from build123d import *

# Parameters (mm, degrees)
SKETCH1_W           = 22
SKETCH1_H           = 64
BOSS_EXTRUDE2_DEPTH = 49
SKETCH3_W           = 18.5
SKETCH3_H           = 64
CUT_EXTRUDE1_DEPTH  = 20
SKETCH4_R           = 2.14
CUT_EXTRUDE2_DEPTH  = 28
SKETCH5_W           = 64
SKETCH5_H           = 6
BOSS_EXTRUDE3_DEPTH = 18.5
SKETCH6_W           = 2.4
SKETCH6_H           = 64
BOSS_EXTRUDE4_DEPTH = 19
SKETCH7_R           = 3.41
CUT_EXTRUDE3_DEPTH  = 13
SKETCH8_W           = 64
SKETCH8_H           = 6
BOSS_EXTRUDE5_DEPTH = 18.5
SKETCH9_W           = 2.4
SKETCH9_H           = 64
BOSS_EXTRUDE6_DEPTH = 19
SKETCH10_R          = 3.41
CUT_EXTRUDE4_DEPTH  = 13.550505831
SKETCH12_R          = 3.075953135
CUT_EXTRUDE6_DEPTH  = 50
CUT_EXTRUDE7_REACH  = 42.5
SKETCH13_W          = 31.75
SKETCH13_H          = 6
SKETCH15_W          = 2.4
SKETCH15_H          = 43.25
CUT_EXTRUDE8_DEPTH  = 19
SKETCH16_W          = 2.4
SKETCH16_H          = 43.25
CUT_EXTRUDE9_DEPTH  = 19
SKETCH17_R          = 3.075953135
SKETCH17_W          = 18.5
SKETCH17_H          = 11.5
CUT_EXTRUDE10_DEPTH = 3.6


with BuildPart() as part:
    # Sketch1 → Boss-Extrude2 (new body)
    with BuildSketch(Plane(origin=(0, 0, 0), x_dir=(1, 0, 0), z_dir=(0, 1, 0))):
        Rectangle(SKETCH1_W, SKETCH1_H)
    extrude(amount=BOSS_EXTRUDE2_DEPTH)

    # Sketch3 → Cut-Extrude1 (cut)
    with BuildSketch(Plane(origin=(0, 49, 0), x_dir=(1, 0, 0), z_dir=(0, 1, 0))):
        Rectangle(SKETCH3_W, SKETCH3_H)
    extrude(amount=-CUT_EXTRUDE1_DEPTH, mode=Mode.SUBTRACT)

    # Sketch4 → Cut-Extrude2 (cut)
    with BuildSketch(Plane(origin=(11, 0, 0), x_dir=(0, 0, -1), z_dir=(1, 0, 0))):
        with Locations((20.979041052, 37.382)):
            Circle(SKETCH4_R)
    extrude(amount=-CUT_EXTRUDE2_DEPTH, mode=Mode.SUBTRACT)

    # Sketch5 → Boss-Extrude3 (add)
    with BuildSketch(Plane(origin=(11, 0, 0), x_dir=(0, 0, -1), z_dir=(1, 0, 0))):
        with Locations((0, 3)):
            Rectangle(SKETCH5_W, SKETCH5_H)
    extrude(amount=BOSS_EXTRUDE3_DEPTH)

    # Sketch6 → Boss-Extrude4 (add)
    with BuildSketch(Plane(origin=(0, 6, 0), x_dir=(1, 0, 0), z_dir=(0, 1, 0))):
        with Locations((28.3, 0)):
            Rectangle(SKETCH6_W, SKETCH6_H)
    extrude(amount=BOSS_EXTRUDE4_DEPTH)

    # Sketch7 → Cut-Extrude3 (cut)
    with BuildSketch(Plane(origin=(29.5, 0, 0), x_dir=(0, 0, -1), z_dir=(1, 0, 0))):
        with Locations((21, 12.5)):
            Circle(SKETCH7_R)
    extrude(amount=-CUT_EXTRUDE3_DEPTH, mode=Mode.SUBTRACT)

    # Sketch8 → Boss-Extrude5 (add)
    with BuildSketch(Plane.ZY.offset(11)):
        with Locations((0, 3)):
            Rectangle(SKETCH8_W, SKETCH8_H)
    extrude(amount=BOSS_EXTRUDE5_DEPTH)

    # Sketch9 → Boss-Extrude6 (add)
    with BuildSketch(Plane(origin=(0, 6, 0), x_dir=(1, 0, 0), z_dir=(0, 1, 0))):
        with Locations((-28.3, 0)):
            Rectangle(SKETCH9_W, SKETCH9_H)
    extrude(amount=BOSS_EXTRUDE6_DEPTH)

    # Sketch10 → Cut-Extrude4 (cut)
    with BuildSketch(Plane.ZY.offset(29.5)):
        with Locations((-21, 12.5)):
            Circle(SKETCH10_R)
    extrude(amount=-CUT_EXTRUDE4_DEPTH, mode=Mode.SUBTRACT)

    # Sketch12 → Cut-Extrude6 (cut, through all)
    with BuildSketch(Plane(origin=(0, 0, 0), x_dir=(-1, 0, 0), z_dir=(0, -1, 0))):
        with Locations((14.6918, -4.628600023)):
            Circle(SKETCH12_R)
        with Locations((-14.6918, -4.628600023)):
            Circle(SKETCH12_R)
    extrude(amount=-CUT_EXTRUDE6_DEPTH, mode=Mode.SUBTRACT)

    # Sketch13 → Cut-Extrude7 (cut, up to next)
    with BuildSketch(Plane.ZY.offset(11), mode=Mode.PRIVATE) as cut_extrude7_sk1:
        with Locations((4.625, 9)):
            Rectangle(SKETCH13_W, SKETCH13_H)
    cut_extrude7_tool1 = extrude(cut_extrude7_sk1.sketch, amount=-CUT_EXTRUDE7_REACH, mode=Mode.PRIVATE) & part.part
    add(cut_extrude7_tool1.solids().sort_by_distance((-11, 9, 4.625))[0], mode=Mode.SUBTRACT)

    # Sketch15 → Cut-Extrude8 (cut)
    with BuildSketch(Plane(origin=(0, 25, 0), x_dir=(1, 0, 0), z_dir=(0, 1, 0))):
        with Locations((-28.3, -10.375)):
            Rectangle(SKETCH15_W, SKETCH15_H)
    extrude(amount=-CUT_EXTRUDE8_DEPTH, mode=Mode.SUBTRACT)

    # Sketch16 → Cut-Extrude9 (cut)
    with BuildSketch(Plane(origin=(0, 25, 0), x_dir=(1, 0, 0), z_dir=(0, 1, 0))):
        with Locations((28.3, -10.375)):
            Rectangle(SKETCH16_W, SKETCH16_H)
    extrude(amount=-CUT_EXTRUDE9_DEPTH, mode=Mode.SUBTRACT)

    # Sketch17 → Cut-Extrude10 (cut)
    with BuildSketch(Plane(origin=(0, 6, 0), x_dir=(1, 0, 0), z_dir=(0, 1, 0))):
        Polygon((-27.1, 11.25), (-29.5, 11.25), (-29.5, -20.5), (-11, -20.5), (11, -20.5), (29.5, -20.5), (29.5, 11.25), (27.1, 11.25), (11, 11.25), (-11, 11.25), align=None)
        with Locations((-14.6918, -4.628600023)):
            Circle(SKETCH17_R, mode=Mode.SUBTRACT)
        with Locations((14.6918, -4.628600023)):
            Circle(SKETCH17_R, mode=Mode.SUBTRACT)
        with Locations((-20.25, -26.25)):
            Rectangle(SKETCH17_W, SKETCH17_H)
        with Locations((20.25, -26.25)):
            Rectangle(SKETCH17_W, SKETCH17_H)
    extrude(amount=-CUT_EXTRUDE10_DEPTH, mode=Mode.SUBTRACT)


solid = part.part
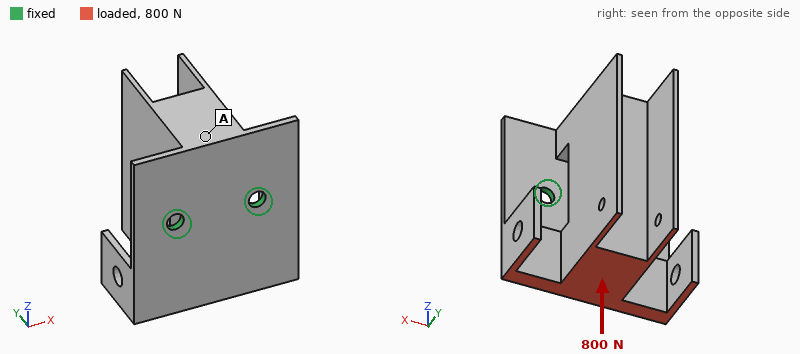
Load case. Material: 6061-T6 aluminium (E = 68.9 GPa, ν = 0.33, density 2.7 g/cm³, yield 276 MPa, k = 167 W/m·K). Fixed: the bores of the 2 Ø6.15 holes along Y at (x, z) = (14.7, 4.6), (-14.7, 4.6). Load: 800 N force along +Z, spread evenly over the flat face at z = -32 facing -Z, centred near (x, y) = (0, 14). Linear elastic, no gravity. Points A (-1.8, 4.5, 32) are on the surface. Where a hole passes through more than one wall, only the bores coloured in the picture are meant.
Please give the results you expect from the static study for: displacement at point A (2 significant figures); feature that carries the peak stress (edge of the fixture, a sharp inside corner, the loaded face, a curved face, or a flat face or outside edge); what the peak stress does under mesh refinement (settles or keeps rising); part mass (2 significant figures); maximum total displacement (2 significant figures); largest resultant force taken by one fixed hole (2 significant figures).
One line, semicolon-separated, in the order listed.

0.15 mm; edge of the fixture; keeps rising; 130 g; 0.32 mm; 400 N
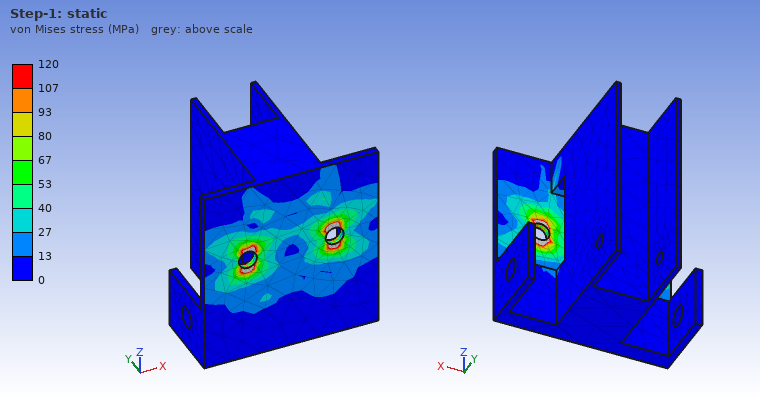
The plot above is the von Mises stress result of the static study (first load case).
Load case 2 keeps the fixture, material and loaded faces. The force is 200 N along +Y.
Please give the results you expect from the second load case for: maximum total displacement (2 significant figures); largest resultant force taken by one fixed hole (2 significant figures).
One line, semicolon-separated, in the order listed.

0.23 mm; 100 N
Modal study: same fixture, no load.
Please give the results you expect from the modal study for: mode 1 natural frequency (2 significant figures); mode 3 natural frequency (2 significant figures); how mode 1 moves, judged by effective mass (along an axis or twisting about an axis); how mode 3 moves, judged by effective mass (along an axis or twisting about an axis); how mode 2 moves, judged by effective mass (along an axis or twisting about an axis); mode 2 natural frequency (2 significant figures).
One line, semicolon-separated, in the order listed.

690 Hz; 2100 Hz; along Z; along Y; along X; 1300 Hz
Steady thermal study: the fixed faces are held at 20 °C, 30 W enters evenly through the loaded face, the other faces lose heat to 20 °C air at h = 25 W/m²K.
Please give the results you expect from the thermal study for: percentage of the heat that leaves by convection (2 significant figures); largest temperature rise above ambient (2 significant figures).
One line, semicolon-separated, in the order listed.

21 %; 19 K
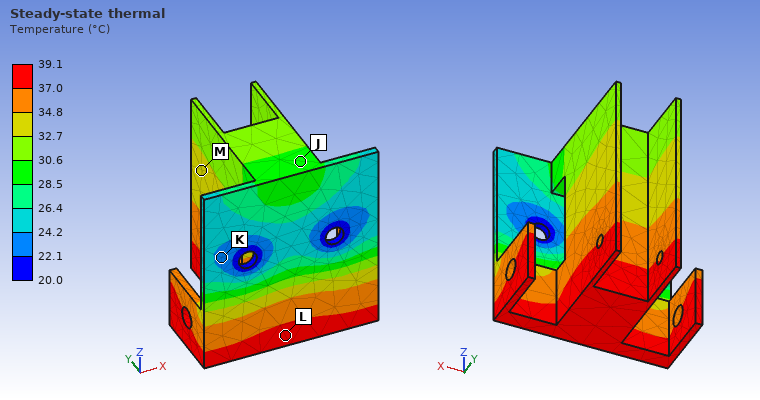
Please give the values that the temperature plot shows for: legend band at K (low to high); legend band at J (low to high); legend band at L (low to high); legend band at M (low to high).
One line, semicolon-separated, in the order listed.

22.1 to 24.2 °C; 28.5 to 30.6 °C; 37.0 to 39.1 °C; 32.7 to 34.8 °C
